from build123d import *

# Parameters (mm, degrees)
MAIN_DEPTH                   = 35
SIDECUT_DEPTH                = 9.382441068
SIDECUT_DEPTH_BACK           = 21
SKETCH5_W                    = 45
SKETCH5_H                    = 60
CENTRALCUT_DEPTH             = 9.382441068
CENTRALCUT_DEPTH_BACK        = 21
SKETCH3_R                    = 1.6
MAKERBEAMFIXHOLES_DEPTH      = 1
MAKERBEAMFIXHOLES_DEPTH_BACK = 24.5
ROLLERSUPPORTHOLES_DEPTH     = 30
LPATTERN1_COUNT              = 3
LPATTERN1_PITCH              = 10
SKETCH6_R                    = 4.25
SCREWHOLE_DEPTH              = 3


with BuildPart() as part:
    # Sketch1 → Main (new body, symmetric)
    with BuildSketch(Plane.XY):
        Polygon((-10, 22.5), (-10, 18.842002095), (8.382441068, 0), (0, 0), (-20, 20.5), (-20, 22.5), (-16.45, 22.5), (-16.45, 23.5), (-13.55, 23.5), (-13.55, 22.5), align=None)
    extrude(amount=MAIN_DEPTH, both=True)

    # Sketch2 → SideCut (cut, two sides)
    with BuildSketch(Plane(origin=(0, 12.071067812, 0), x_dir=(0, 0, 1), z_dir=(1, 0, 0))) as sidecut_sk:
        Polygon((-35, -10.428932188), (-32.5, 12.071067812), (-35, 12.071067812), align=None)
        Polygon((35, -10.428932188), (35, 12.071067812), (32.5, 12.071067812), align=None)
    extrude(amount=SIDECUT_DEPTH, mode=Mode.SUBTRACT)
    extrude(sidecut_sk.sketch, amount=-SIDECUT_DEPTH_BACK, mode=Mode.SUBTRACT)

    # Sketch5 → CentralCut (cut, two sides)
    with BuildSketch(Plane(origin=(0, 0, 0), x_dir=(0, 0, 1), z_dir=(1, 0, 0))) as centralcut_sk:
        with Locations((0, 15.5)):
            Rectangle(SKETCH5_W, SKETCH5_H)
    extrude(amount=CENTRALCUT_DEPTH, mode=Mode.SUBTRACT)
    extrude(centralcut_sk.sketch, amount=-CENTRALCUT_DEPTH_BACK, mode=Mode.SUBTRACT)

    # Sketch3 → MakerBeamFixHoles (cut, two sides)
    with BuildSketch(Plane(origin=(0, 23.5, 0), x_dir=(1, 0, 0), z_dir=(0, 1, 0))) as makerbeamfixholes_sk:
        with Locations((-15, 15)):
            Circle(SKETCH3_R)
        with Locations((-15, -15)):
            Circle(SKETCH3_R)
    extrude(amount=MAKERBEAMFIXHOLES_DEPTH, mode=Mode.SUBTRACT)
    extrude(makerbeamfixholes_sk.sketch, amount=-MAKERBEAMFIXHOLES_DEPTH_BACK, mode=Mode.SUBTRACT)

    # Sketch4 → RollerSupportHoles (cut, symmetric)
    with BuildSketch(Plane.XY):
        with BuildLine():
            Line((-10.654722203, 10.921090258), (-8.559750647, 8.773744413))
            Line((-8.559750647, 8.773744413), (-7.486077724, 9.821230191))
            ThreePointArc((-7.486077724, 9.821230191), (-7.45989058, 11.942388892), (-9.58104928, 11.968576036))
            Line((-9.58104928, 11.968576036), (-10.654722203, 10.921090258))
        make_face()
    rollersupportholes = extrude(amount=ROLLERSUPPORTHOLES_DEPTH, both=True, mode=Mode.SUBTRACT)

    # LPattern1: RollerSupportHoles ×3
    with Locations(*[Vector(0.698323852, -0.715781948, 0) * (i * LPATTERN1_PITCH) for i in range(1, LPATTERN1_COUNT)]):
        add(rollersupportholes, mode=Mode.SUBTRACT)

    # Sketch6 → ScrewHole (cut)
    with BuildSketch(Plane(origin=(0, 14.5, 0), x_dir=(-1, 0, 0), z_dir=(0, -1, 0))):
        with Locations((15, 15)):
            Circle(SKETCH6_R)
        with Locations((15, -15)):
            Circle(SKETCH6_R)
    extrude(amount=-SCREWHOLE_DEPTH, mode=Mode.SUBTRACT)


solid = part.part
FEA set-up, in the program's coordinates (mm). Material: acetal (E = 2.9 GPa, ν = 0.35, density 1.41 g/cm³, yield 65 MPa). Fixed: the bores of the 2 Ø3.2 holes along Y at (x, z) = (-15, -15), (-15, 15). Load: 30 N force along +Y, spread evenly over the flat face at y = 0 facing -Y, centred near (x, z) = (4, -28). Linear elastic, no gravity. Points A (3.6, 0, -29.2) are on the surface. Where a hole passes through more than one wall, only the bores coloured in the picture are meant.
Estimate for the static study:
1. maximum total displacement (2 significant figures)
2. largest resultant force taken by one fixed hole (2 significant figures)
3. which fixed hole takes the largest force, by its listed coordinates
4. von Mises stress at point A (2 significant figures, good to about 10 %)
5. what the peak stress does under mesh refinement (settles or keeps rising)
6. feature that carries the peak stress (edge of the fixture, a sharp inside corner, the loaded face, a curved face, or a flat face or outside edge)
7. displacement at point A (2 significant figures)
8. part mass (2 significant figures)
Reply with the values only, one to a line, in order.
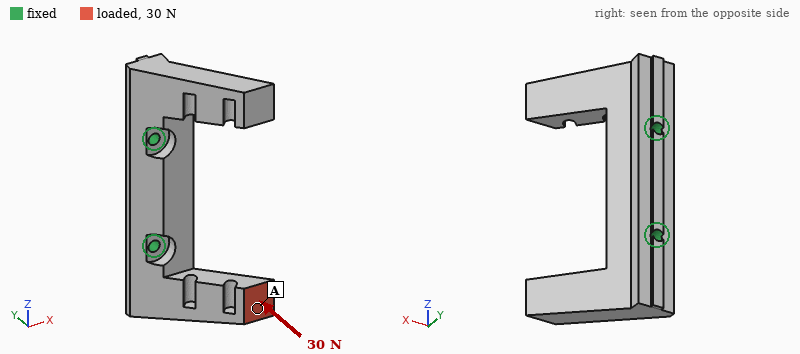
0.73 mm
36 N
(-15, -15)
1.8 MPa
keeps rising
edge of the fixture
0.61 mm
10 g
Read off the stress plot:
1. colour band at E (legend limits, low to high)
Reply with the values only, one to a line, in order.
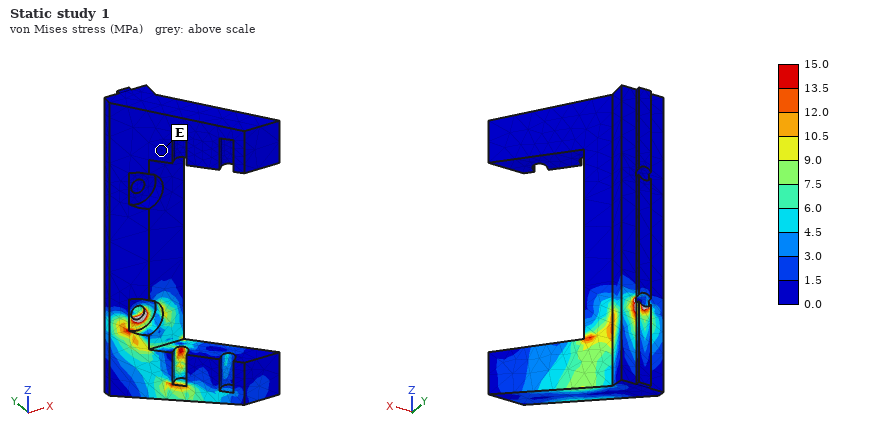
0.0 to 1.5 MPa
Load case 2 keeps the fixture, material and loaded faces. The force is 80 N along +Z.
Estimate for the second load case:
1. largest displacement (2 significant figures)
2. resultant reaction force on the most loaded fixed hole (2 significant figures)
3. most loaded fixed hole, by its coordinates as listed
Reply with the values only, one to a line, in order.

0.87 mm
84 N
(-15, 15)
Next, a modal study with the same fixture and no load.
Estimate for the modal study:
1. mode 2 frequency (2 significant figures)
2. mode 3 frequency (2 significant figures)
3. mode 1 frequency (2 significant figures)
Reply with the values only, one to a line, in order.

1100 Hz
1900 Hz
1100 Hz
